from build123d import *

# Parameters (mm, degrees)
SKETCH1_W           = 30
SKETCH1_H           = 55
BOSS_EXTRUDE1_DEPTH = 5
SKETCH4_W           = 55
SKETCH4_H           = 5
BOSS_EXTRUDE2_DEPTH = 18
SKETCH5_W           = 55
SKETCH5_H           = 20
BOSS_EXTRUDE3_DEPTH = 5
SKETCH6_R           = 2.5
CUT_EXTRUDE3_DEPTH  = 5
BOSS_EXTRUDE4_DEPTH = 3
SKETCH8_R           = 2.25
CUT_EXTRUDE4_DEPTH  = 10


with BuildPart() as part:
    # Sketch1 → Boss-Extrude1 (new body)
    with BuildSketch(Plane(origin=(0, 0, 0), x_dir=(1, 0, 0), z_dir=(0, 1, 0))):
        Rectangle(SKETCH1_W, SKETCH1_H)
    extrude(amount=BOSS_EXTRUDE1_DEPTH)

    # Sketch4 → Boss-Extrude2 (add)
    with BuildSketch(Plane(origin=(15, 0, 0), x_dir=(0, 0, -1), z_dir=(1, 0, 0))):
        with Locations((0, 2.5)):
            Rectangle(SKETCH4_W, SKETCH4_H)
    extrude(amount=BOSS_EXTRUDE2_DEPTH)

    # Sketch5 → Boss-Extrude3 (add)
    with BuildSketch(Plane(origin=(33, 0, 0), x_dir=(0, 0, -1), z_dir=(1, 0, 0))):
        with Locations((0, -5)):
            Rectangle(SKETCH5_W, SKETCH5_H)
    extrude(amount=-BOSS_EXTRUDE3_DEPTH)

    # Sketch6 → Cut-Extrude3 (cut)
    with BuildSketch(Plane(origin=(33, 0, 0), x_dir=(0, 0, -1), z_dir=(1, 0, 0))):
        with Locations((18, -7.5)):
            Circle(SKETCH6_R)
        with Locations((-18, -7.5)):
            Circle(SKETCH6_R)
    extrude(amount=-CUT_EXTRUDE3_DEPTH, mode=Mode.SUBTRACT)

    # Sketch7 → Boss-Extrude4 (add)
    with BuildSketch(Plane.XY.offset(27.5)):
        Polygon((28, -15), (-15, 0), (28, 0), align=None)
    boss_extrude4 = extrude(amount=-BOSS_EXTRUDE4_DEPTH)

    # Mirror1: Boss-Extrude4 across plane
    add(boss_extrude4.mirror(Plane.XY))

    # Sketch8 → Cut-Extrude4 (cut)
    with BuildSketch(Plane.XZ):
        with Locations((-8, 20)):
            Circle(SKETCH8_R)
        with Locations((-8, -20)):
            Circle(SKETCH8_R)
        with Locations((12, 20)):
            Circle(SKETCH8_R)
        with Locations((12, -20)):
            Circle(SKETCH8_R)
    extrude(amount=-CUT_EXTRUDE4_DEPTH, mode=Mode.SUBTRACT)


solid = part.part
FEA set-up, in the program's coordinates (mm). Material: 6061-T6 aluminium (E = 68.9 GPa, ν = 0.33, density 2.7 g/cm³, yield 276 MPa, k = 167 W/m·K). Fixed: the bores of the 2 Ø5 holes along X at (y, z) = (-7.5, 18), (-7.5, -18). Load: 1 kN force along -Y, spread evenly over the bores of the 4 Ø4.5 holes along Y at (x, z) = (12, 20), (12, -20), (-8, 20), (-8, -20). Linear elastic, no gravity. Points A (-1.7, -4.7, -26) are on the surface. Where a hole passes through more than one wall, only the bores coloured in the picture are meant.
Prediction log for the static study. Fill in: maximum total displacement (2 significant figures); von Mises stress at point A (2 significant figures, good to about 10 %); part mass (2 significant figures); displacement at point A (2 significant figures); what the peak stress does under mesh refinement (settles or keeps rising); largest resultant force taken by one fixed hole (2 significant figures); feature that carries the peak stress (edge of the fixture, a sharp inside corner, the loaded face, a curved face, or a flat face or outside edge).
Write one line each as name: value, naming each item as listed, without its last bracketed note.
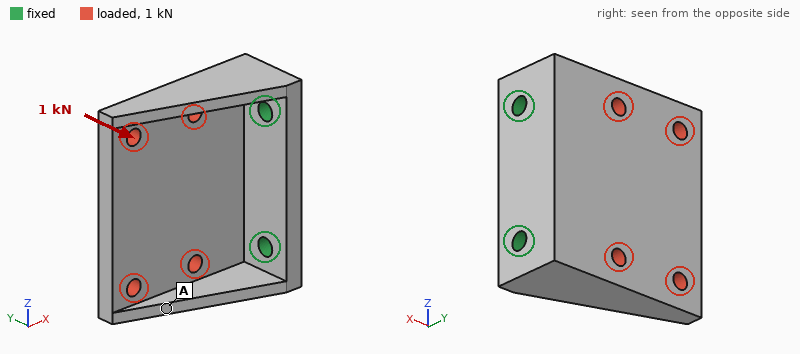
maximum total displacement: 0.24 mm
von Mises stress at point A: 29 MPa
part mass: 51 g
displacement at point A: 0.14 mm
what the peak stress does under mesh refinement: keeps rising
largest resultant force taken by one fixed hole: 500 N
feature that carries the peak stress: edge of the fixture
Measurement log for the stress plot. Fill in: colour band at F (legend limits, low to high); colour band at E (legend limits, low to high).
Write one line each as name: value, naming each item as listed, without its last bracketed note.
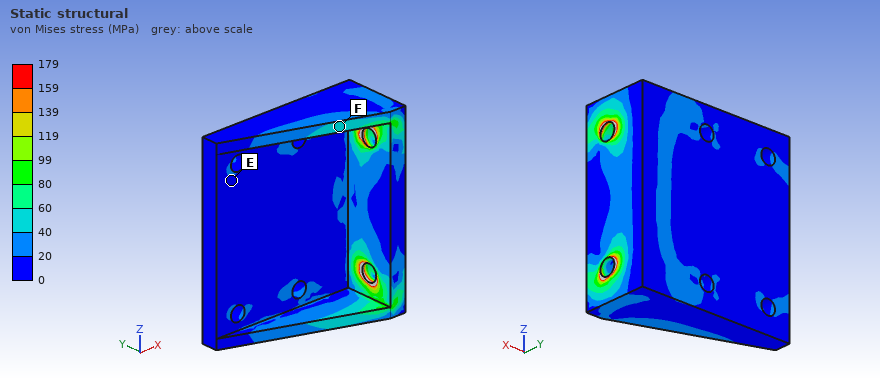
colour band at F: 40 to 60 MPa
colour band at E: 0 to 20 MPa
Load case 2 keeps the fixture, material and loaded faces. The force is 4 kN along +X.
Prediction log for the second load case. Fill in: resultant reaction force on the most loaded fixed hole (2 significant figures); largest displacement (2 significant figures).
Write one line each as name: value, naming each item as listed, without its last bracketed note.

resultant reaction force on the most loaded fixed hole: 2.0 kN
largest displacement: 0.20 mm
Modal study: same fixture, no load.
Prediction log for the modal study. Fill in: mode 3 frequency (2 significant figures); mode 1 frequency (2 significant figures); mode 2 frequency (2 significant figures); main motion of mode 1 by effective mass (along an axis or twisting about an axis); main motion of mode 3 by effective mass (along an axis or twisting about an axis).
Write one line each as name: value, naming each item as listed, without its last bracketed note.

mode 3 frequency: 8200 Hz
mode 1 frequency: 2400 Hz
mode 2 frequency: 4000 Hz
main motion of mode 1 by effective mass: along Y
main motion of mode 3 by effective mass: along Z
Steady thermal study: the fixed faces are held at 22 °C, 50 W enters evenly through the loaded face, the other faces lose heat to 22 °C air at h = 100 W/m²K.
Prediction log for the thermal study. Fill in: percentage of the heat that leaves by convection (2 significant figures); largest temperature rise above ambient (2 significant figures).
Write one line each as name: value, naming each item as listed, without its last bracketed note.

percentage of the heat that leaves by convection: 28 %
largest temperature rise above ambient: 31 K
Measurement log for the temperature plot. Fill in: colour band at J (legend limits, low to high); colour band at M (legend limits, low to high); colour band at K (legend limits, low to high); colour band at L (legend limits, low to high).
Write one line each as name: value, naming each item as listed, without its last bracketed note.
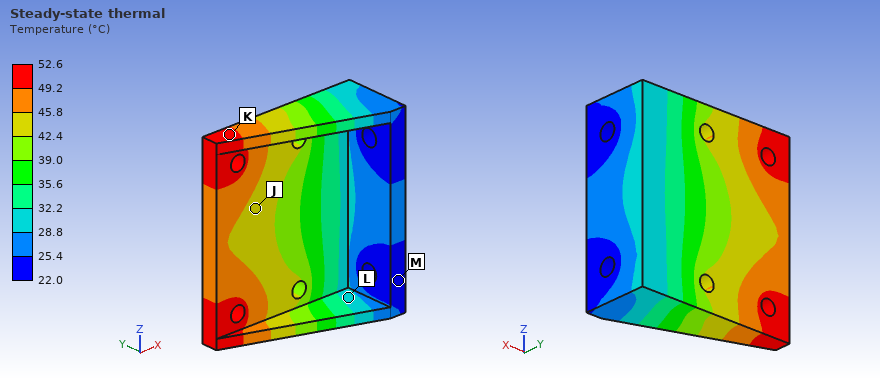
colour band at J: 42.4 to 45.8 °C
colour band at M: 22.0 to 25.4 °C
colour band at K: 49.2 to 52.6 °C
colour band at L: 28.8 to 32.2 °C
